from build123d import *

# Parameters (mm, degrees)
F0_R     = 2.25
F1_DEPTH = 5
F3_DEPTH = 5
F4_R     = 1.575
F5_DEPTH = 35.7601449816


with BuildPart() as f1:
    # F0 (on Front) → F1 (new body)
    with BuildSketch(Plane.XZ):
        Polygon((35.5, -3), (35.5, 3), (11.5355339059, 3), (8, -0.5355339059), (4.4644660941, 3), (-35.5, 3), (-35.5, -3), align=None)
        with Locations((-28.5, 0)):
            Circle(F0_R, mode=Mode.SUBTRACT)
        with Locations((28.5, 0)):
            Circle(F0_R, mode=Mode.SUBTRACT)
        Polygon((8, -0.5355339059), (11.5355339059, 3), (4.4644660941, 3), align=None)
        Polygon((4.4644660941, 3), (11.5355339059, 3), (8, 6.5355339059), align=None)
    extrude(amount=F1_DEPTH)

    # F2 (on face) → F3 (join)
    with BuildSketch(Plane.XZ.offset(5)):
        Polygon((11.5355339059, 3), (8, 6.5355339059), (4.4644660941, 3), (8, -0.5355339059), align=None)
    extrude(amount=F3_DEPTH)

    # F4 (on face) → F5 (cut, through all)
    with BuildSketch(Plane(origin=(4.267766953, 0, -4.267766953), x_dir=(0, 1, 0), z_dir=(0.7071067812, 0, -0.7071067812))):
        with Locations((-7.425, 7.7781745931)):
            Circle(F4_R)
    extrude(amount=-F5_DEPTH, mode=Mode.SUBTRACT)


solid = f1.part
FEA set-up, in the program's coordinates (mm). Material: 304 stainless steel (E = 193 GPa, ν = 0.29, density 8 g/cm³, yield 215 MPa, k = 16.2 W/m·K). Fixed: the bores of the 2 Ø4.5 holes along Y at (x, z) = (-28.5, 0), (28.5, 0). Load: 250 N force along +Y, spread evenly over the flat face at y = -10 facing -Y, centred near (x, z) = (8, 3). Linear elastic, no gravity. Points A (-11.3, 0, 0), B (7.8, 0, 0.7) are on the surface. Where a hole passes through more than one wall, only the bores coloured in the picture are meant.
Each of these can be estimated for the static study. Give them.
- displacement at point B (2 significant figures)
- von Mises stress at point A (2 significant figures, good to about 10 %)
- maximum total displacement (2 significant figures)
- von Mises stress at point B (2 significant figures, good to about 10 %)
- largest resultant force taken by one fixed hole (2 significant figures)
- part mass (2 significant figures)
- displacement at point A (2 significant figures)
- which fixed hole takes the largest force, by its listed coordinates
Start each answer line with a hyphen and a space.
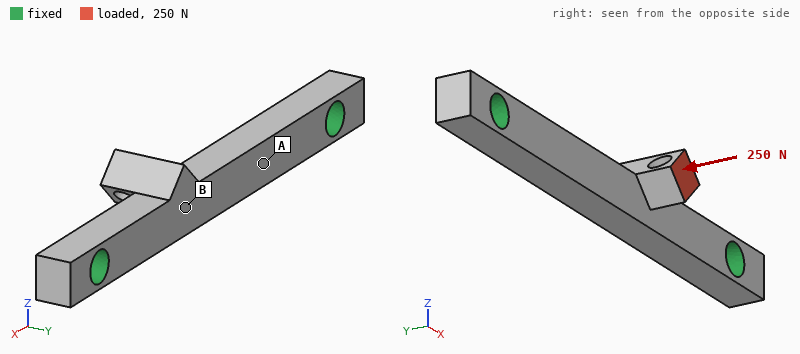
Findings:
- 14 µm
- 13 MPa
- 21 µm
- 44 MPa
- 180 N
- 17 g
- 7.7 µm
- (28.5, 0)
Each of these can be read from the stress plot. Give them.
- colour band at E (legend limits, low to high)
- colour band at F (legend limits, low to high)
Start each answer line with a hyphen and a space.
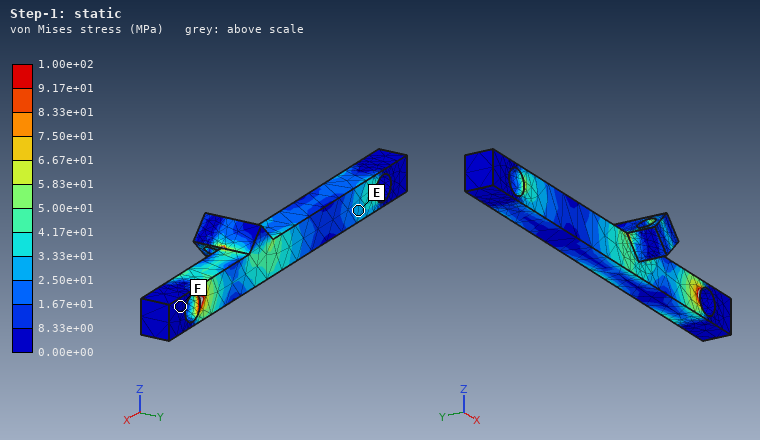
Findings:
- 2.50e+01 to 3.33e+01 MPa
- 0.00e+00 to 8.33e+00 MPa
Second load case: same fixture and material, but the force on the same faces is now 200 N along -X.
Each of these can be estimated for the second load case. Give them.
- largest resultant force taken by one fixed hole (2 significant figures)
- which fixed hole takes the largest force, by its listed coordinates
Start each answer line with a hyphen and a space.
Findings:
- 140 N
- (28.5, 0)
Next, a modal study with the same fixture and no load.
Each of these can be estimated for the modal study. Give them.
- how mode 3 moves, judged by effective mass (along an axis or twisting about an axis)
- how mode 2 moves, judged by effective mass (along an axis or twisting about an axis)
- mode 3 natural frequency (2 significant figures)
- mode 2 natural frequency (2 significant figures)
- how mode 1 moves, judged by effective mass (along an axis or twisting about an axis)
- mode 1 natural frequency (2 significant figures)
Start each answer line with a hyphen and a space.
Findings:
- twisting about X
- along Z
- 18 kHz
- 8800 Hz
- along Y
- 7800 Hz
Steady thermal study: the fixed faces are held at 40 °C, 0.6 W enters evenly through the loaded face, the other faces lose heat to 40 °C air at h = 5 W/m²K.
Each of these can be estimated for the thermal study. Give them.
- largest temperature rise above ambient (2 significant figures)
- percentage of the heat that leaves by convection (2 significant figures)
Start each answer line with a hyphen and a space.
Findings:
- 30 K
- 9.3 %
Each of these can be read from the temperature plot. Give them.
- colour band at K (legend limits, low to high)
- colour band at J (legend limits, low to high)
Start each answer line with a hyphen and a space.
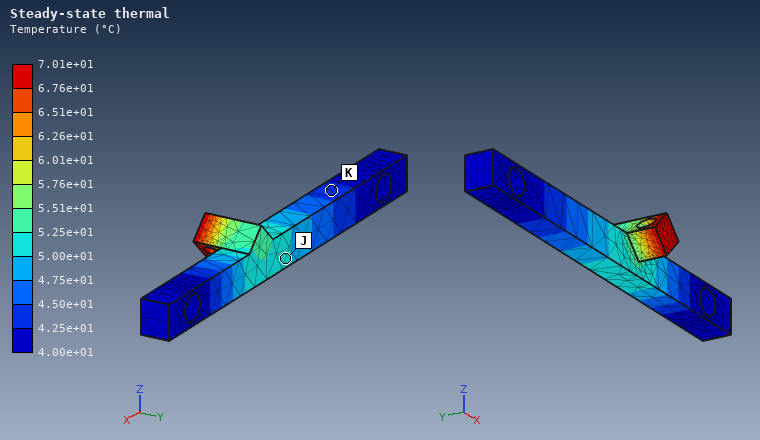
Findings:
- 4.25e+01 to 4.50e+01 °C
- 5.00e+01 to 5.25e+01 °C
